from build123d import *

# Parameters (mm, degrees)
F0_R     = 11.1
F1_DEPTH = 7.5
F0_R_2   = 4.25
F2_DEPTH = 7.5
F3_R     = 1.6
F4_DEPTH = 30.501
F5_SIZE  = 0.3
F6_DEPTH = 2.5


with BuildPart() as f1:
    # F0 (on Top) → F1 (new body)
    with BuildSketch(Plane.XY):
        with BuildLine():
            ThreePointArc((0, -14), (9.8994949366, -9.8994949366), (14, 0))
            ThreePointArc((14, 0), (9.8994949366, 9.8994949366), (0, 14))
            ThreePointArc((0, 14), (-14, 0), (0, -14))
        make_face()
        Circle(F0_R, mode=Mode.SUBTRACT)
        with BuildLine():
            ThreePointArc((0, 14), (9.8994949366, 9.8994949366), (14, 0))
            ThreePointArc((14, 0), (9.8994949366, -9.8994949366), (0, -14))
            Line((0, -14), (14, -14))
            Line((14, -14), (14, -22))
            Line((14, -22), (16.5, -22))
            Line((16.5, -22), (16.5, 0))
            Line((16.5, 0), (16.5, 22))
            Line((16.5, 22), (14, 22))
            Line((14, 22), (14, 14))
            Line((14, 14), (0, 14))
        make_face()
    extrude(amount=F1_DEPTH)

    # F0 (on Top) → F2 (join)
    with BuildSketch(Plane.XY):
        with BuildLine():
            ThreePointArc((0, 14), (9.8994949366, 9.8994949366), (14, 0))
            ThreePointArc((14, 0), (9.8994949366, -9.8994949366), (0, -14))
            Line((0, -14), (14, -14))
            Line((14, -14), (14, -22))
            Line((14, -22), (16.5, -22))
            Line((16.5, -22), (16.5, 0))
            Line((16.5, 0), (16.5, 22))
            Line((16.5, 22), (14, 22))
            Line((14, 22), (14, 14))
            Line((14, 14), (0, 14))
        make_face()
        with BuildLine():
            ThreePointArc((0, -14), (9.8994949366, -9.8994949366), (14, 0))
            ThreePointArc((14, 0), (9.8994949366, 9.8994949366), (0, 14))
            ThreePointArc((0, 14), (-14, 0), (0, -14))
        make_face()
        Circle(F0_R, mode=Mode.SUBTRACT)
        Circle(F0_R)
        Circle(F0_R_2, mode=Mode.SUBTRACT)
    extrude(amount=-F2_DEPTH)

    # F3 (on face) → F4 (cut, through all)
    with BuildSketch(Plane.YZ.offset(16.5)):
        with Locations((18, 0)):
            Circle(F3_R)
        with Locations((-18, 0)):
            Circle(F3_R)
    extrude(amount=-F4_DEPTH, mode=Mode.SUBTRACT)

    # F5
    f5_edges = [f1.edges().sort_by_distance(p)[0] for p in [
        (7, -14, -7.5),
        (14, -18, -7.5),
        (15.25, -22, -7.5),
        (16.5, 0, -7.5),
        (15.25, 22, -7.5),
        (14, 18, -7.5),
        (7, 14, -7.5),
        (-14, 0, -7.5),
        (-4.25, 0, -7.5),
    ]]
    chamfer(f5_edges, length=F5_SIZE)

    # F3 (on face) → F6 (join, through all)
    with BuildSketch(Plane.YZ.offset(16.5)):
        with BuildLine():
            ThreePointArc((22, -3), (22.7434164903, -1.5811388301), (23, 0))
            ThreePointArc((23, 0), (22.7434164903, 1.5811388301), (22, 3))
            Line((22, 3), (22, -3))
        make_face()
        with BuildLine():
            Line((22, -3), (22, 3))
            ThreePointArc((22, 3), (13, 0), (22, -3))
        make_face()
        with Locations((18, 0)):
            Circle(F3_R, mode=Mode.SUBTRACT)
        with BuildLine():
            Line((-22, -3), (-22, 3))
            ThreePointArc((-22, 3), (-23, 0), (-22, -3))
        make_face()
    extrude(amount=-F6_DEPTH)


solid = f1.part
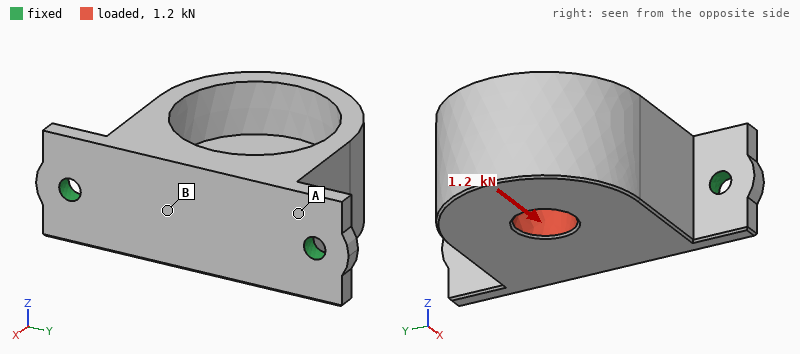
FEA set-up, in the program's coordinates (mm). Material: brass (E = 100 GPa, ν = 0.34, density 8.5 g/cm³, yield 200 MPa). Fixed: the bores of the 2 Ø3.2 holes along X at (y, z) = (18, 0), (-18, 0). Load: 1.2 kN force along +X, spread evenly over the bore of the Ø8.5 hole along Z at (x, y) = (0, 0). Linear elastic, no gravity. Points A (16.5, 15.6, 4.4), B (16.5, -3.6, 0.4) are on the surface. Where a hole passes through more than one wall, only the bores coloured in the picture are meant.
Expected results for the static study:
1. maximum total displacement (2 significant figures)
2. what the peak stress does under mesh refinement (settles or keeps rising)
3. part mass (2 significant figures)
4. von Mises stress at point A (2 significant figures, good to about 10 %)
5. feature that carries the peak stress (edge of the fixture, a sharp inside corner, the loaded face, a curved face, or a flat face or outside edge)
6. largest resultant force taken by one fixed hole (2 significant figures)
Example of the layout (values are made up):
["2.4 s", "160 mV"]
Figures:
["80 µm", "keeps rising", "75 g", "40 MPa", "edge of the fixture", "680 N"]
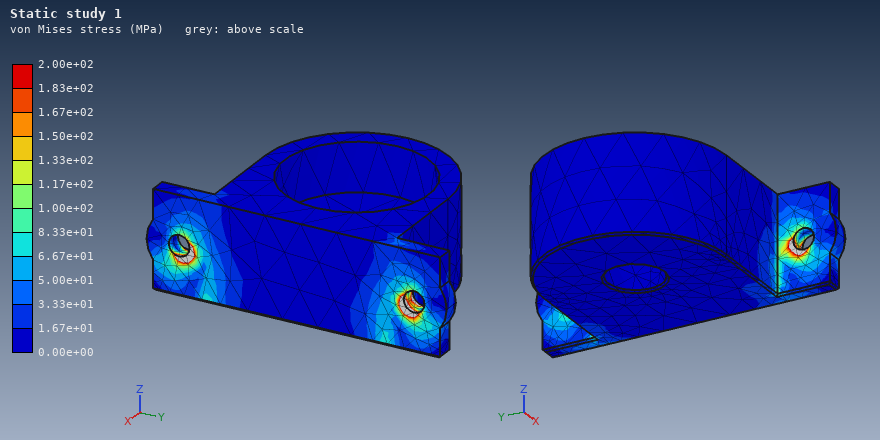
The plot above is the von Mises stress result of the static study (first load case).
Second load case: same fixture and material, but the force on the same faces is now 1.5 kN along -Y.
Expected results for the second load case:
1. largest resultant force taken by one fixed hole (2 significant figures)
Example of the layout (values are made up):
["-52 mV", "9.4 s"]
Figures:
["1.1 kN"]
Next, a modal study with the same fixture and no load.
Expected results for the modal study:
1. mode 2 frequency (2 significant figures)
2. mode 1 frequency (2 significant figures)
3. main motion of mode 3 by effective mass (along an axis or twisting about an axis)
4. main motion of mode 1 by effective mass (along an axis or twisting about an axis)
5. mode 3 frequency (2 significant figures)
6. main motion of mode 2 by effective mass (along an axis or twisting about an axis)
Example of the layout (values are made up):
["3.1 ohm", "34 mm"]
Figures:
["6200 Hz", "1600 Hz", "along X", "along Z", "7400 Hz", "along Y"]
